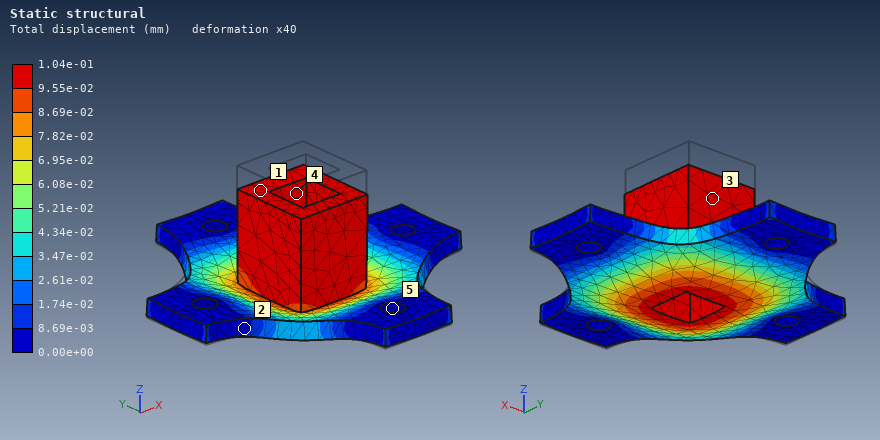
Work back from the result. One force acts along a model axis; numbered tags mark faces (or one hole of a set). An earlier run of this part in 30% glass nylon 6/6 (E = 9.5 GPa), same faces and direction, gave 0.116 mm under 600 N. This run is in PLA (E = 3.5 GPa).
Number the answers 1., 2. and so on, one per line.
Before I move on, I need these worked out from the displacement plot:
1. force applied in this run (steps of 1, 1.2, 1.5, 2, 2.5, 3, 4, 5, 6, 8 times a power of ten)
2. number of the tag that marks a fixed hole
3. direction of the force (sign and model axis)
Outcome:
1. 200 N
2. 5
3. -Z
